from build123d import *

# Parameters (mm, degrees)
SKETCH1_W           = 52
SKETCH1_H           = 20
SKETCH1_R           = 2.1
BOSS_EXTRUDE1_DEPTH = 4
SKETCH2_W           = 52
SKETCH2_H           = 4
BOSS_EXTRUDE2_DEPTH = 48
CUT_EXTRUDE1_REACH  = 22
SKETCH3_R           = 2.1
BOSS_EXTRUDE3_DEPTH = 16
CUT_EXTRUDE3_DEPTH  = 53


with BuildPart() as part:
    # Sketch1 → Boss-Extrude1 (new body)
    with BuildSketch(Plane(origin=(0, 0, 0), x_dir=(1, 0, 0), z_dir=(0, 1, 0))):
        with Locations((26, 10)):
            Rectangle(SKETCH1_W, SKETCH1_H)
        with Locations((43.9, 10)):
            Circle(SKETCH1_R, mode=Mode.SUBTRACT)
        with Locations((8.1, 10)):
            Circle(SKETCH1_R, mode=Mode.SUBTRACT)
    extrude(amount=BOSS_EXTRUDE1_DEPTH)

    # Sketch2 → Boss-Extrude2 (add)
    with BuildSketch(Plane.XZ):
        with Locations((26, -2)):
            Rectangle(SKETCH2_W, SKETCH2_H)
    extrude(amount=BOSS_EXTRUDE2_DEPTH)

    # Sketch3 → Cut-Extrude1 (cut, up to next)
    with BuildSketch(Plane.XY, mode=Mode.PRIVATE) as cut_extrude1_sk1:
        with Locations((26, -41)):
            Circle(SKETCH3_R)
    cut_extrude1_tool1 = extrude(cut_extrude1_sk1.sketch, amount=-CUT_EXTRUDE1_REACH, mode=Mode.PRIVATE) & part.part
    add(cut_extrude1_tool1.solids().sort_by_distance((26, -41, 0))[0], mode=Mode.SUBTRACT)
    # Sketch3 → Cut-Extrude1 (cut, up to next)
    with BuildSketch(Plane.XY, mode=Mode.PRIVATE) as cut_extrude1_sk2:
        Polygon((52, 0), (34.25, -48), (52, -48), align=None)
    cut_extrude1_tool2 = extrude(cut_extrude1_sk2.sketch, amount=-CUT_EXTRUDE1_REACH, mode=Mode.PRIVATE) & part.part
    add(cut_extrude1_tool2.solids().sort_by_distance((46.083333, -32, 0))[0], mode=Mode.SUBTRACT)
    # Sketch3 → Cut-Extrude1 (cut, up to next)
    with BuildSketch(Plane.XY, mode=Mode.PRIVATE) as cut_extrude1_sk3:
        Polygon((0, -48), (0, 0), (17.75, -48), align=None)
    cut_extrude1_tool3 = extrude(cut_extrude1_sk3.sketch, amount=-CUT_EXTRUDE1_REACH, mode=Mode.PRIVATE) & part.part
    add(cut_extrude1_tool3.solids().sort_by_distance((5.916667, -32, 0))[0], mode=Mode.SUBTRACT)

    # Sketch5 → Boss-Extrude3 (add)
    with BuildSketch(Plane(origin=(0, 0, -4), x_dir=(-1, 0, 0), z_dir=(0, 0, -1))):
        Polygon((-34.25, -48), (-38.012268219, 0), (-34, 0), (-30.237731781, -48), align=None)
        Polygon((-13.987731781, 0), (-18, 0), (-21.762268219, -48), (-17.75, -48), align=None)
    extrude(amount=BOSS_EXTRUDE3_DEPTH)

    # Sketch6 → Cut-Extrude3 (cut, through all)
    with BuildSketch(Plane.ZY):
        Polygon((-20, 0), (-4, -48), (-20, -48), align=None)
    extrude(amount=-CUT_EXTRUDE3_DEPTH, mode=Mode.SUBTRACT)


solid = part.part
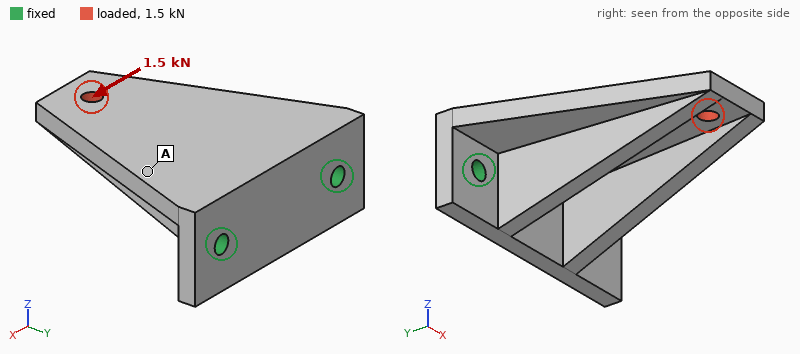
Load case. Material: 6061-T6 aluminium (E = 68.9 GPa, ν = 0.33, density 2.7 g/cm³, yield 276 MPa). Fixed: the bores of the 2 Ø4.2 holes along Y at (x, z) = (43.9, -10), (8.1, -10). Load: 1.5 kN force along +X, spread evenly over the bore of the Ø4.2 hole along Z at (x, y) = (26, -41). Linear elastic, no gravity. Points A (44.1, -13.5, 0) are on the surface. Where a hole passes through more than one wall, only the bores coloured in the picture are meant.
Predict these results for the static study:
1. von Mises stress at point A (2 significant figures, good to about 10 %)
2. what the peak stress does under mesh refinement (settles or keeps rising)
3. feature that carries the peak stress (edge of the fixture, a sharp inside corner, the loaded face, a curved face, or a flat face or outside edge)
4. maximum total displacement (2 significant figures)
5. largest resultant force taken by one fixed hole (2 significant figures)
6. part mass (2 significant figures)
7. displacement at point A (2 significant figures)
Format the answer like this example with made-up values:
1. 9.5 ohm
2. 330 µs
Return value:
1. 23 MPa
2. keeps rising
3. edge of the fixture
4. 0.11 mm
5. 2.0 kN
6. 37 g
7. 0.041 mm
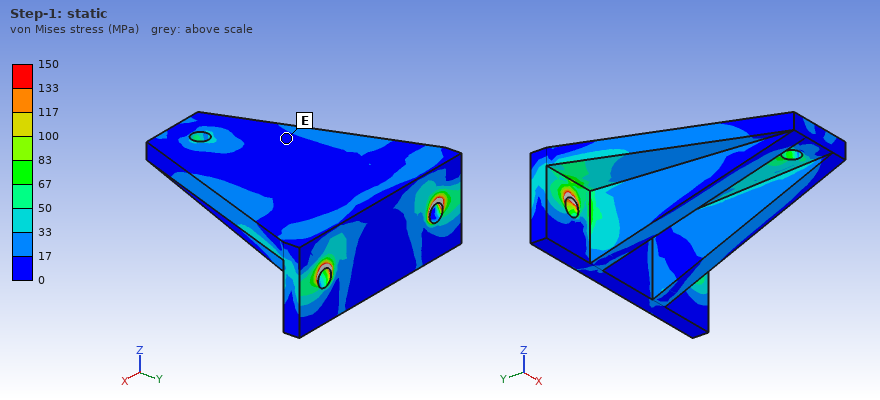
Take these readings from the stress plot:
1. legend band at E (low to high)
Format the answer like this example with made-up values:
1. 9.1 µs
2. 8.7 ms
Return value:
1. 0 to 17 MPa
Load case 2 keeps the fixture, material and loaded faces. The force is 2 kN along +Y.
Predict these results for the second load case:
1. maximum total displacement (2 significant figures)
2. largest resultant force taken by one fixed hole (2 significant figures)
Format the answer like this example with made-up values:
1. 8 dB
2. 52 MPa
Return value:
1. 0.16 mm
2. 1.0 kN
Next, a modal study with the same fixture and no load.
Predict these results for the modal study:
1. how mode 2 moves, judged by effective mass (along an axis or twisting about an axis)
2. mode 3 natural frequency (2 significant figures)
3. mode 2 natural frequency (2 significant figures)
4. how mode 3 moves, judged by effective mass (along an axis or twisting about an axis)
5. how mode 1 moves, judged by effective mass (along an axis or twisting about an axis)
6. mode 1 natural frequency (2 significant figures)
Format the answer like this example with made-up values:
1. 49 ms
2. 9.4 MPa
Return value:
1. along X
2. 9600 Hz
3. 6000 Hz
4. along X
5. along Z
6. 2600 Hz
